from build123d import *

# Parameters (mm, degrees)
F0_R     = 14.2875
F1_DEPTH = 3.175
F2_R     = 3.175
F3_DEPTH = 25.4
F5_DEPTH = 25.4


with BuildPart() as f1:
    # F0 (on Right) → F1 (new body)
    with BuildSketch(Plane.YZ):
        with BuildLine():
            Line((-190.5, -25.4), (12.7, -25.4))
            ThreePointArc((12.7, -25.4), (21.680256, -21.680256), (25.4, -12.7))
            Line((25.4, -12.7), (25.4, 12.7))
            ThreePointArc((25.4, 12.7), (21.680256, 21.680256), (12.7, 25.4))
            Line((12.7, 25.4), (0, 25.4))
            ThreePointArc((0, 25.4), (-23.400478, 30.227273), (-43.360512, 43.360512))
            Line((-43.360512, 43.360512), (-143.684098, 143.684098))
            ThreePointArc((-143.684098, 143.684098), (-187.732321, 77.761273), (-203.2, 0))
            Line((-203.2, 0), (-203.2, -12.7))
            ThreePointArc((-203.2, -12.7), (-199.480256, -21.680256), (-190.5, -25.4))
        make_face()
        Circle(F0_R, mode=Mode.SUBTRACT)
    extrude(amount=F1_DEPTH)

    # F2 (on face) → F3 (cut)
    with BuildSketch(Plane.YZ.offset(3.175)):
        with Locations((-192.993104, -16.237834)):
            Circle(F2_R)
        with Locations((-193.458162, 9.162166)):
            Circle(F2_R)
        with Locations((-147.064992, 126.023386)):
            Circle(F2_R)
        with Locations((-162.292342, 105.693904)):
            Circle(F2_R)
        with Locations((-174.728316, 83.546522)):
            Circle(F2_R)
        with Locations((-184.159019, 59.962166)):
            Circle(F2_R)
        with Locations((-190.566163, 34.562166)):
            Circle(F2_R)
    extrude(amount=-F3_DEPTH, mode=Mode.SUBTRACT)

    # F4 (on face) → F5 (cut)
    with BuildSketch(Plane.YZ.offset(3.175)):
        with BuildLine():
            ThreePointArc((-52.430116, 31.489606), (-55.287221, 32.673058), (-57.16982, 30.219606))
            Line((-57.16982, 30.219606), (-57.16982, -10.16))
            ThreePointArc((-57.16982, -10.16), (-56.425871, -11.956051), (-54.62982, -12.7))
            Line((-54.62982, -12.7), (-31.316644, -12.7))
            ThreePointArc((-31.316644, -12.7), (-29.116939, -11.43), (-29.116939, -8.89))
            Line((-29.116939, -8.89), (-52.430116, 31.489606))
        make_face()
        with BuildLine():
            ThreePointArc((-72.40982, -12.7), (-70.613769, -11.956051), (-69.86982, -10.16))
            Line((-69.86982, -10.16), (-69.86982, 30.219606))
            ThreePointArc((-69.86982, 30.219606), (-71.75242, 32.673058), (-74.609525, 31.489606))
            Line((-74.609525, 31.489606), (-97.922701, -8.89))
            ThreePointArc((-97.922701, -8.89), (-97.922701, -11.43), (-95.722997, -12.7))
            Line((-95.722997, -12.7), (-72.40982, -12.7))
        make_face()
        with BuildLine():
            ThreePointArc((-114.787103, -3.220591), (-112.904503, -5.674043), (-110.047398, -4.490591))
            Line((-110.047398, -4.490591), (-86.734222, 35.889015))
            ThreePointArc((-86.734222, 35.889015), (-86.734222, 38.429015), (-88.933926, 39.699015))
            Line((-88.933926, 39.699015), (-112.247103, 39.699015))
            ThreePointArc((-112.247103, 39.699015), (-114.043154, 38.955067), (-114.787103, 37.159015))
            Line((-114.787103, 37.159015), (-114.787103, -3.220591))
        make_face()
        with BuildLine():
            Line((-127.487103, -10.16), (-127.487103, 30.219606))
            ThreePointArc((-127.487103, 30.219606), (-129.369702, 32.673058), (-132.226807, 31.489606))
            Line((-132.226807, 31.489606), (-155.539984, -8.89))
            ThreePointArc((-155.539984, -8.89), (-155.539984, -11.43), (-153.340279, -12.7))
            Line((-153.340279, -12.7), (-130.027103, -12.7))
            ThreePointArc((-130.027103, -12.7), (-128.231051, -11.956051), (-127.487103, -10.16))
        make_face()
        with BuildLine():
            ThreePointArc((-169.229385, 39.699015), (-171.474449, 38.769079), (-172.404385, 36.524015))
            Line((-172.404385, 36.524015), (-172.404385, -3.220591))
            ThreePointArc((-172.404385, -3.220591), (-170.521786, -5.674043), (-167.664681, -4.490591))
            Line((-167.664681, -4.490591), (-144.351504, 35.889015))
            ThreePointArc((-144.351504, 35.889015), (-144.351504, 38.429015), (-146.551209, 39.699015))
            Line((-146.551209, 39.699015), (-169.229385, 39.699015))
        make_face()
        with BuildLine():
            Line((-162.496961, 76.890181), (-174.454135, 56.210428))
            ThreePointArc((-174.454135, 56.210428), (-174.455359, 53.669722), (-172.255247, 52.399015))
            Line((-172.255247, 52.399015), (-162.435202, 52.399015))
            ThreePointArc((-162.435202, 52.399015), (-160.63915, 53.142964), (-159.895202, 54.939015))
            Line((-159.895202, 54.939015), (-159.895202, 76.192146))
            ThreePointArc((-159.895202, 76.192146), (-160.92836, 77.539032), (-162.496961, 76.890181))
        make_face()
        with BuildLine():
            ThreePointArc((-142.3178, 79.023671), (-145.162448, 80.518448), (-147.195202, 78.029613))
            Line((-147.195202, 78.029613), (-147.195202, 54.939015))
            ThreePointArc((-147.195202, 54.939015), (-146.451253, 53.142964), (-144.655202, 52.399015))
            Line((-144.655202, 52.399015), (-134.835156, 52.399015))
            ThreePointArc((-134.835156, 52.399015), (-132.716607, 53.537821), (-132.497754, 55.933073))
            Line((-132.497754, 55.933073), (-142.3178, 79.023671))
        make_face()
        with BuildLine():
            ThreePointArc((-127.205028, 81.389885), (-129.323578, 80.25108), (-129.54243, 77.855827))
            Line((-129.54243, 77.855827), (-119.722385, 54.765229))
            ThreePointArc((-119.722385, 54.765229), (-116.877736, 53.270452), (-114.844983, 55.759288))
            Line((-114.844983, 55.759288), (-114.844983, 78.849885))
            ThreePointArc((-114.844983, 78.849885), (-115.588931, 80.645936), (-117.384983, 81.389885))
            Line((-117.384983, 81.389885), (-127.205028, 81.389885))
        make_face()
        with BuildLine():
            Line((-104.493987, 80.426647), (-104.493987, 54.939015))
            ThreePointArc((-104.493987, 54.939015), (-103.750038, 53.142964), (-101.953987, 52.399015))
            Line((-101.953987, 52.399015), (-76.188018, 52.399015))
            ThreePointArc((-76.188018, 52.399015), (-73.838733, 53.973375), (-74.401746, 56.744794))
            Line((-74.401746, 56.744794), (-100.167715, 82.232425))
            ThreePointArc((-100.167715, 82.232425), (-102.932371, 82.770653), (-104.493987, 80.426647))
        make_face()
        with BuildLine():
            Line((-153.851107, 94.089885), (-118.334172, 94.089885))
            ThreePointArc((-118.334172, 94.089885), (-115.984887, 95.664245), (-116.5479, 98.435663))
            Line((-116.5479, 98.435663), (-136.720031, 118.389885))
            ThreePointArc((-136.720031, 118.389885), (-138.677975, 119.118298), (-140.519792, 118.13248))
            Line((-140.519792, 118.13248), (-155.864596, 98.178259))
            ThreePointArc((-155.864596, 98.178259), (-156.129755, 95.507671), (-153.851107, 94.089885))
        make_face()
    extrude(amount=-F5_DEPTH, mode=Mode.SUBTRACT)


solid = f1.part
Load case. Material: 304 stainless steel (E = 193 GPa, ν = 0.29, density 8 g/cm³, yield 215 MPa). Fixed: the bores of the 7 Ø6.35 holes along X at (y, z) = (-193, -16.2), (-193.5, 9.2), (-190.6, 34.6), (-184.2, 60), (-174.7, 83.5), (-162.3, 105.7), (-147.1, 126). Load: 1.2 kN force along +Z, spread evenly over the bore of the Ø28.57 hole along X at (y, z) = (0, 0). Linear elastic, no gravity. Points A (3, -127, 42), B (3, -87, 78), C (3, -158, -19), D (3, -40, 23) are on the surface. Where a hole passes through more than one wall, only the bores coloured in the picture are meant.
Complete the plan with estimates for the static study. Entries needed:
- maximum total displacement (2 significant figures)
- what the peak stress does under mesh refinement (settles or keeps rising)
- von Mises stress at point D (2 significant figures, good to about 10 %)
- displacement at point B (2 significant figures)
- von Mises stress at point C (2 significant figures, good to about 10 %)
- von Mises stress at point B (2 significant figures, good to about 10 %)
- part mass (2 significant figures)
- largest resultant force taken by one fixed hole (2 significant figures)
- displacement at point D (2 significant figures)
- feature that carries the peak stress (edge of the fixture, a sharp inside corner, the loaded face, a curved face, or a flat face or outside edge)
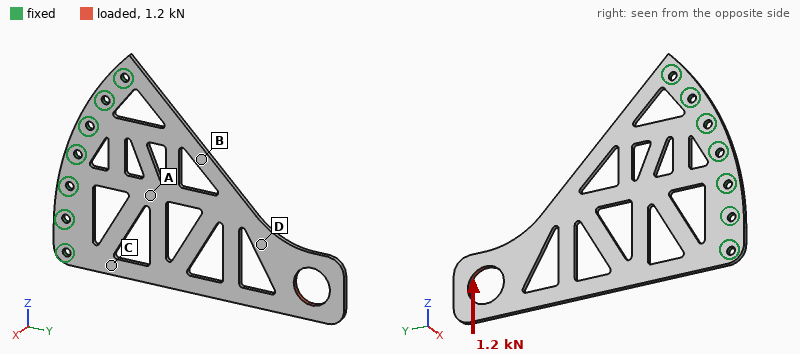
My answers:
84 µm
keeps rising
21 MPa
16 µm
28 MPa
34 MPa
410 g
1.3 kN
38 µm
edge of the fixture
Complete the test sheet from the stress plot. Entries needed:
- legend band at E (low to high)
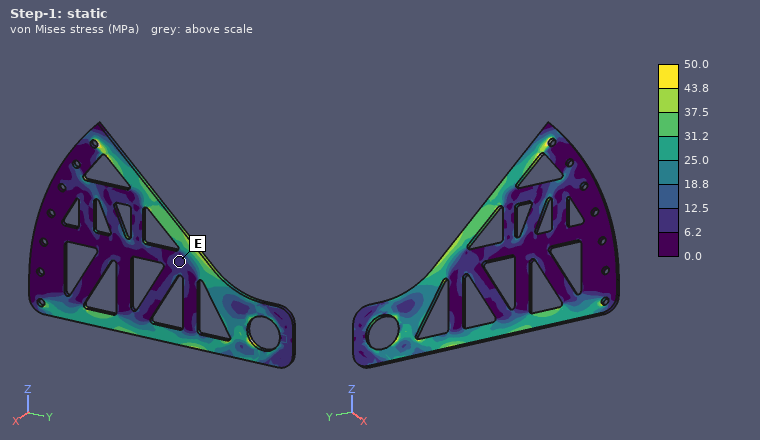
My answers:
6.2 to 12.5 MPa
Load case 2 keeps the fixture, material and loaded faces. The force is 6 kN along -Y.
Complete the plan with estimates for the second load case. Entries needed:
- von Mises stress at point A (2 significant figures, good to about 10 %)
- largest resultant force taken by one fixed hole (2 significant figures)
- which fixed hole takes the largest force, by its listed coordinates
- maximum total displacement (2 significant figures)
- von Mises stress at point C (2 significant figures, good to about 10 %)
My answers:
24 MPa
3.8 kN
(-193, -16.2)
0.13 mm
91 MPa
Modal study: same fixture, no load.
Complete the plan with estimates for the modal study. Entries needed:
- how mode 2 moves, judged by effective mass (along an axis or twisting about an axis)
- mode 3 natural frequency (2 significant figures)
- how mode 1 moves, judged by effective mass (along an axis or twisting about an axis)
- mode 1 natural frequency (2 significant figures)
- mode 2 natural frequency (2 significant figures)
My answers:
along X
410 Hz
along X
71 Hz
330 Hz
